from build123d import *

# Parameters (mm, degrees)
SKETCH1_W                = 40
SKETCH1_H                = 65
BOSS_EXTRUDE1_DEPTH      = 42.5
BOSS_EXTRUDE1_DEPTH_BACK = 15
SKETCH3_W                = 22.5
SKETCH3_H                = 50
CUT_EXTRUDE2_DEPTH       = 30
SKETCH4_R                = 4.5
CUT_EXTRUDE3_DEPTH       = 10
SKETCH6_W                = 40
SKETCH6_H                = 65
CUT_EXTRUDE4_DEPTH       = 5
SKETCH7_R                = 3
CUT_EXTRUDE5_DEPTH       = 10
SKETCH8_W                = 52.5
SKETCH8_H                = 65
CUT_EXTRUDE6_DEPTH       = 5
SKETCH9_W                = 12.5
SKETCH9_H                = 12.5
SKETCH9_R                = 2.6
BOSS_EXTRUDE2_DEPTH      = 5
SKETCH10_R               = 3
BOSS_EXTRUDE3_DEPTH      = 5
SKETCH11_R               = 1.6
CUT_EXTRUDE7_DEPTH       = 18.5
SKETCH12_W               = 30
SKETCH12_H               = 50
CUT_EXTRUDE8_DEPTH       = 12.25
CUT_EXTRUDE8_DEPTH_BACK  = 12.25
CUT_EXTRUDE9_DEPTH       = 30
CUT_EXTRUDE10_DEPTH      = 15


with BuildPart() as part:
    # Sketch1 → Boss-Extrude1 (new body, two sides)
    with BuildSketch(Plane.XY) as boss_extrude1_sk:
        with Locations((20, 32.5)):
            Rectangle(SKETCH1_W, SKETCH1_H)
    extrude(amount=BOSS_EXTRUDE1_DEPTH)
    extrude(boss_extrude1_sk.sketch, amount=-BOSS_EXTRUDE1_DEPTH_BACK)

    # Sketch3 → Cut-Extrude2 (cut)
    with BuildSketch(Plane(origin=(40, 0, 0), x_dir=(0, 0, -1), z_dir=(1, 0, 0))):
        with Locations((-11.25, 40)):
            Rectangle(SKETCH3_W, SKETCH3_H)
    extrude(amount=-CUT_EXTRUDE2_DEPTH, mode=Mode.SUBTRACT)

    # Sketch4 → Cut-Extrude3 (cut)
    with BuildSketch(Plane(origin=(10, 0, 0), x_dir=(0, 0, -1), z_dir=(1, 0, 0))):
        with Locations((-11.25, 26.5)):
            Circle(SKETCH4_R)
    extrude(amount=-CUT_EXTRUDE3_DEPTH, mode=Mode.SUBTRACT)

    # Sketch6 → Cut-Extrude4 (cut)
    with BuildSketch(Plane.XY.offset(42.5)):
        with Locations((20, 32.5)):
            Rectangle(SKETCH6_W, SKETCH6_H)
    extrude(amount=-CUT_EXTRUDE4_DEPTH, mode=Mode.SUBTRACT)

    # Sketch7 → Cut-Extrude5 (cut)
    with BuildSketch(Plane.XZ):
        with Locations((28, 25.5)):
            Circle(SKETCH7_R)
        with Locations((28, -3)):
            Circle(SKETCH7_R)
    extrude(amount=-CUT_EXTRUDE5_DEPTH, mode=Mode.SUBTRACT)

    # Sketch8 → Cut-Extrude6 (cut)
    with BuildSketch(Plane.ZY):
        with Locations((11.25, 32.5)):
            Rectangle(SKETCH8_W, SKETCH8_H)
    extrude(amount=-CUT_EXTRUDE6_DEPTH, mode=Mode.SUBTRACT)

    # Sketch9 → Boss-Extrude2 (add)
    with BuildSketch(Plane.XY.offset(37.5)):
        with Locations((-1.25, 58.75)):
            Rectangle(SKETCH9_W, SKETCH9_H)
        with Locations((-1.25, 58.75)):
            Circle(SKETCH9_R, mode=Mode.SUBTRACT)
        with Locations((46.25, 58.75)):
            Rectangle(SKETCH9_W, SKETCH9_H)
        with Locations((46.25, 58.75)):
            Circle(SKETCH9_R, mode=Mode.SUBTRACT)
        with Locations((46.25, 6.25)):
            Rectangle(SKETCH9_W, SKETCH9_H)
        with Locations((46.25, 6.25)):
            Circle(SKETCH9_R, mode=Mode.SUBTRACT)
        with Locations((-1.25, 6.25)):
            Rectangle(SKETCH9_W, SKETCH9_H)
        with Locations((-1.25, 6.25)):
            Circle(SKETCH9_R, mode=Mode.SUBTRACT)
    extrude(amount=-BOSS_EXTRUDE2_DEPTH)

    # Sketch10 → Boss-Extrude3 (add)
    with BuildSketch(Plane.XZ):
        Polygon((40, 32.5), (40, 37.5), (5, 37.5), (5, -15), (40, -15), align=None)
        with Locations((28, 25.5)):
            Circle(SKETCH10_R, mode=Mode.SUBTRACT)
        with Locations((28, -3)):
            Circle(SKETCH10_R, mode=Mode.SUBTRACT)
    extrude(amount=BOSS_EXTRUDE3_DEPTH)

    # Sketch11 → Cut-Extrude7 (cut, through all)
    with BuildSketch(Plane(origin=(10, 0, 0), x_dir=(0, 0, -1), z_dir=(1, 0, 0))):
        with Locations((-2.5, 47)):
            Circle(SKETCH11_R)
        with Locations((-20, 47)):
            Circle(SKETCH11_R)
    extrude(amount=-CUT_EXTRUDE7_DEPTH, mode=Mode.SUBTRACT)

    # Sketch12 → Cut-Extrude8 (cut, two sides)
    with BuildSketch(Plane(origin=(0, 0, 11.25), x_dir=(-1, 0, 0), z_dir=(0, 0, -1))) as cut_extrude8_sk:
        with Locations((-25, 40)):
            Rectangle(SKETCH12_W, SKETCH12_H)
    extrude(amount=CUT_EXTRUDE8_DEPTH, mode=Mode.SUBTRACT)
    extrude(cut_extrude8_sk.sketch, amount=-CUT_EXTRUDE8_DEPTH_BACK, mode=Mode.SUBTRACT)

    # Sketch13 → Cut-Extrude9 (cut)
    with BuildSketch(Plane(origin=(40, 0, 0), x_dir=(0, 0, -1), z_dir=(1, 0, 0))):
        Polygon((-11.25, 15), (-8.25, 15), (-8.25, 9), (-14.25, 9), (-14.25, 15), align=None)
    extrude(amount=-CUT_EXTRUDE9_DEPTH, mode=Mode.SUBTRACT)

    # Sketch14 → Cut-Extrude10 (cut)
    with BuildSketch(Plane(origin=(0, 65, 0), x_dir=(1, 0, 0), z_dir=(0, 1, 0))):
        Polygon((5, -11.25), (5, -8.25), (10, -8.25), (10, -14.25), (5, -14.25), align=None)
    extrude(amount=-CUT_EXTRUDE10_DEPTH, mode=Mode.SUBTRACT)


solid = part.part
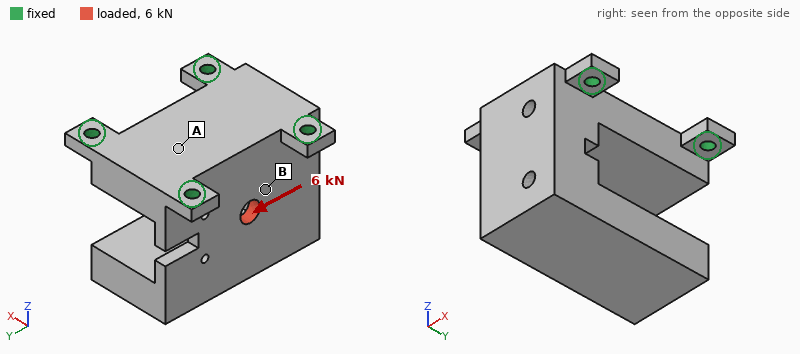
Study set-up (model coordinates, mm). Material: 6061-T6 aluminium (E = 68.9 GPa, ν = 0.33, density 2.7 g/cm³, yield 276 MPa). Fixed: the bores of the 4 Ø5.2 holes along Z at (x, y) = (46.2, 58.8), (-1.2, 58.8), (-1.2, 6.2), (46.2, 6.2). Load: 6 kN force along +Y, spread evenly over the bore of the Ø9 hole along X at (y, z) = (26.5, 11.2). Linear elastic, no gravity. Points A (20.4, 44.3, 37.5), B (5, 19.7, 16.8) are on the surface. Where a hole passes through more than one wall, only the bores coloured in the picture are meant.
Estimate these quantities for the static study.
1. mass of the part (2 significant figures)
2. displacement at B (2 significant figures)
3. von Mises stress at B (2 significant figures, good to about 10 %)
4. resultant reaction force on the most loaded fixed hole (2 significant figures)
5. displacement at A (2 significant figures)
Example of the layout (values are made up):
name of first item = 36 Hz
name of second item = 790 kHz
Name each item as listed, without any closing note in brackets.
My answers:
mass of the part = 250 g
displacement at B = 33 µm
von Mises stress at B = 36 MPa
resultant reaction force on the most loaded fixed hole = 2.5 kN
displacement at A = 14 µm
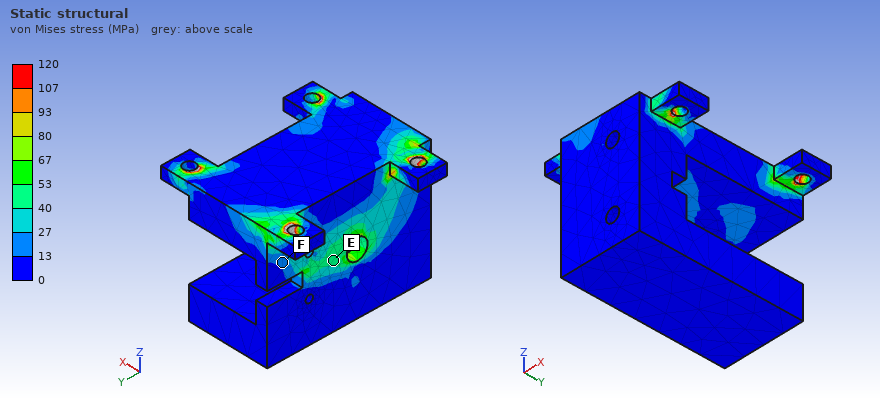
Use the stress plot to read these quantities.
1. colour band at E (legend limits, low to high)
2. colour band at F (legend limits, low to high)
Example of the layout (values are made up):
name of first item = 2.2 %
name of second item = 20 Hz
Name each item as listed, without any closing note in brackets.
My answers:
colour band at E = 40 to 53 MPa
colour band at F = 13 to 27 MPa
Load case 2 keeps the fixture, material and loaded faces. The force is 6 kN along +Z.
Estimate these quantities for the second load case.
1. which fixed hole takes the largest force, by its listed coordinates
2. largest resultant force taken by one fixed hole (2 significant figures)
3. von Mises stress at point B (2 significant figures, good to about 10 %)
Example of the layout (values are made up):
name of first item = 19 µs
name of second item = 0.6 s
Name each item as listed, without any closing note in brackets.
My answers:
which fixed hole takes the largest force, by its listed coordinates = (-1.2, 6.2)
largest resultant force taken by one fixed hole = 3.3 kN
von Mises stress at point B = 29 MPa
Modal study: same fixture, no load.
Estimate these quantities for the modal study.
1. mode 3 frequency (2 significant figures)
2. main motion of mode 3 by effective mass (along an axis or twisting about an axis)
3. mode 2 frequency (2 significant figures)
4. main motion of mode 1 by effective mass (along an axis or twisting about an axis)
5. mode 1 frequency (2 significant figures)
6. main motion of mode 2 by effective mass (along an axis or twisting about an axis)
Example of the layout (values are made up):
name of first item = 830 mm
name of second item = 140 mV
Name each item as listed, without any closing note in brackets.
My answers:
mode 3 frequency = 4900 Hz
main motion of mode 3 by effective mass = along Z
mode 2 frequency = 2900 Hz
main motion of mode 1 by effective mass = along X
mode 1 frequency = 2400 Hz
main motion of mode 2 by effective mass = along Y
